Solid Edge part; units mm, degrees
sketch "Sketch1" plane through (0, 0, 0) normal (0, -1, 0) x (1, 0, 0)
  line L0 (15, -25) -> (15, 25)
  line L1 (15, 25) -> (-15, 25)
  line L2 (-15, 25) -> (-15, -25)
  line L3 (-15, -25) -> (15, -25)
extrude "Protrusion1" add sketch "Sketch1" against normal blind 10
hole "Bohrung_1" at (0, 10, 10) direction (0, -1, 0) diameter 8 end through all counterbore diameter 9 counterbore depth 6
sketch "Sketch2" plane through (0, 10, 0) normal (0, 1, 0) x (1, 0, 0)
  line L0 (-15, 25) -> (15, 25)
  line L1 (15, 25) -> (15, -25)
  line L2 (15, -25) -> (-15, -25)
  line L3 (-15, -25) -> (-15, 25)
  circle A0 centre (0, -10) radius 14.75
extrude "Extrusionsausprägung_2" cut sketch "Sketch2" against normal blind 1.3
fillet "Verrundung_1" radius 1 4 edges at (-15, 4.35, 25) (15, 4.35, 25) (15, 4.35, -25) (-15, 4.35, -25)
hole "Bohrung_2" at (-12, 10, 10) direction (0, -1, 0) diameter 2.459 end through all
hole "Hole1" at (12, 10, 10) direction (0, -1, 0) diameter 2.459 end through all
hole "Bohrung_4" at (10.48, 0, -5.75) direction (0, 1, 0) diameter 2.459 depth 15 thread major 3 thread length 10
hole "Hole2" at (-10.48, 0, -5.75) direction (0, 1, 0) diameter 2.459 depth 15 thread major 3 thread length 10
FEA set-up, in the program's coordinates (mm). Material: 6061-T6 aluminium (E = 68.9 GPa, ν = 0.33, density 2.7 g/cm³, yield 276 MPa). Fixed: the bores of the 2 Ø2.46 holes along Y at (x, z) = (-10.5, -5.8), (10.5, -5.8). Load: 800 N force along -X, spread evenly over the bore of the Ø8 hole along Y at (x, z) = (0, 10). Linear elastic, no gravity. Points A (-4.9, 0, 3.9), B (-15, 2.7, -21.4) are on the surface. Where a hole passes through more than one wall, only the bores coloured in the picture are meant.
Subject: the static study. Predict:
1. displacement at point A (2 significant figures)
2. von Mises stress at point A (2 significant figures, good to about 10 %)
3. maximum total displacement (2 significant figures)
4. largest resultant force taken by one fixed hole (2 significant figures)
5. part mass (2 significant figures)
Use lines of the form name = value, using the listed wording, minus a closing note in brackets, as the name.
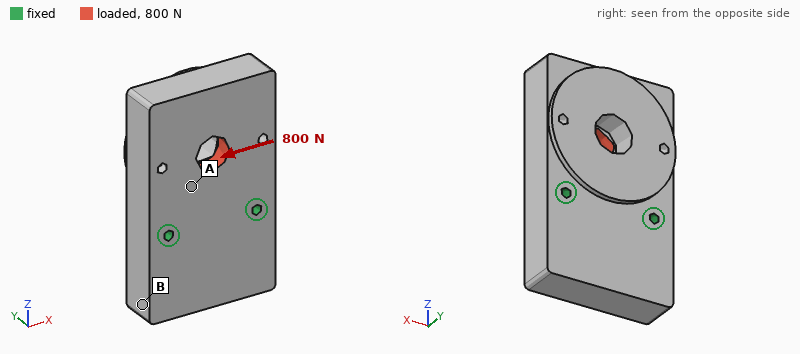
displacement at point A = 2.2 µm
von Mises stress at point A = 9.7 MPa
maximum total displacement = 6.8 µm
largest resultant force taken by one fixed hole = 700 N
part mass = 36 g
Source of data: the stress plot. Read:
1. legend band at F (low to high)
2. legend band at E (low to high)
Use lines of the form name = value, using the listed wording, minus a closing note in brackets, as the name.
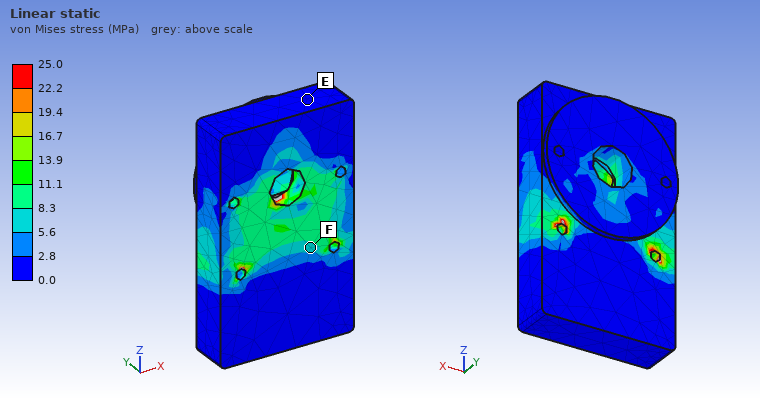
legend band at F = 5.6 to 8.3 MPa
legend band at E = 0.0 to 2.8 MPa
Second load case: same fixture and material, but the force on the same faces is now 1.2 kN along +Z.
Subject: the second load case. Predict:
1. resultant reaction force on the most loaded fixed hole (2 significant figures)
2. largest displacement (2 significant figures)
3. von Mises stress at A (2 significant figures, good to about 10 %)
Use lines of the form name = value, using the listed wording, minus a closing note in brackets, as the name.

resultant reaction force on the most loaded fixed hole = 610 N
largest displacement = 11 µm
von Mises stress at A = 13 MPa
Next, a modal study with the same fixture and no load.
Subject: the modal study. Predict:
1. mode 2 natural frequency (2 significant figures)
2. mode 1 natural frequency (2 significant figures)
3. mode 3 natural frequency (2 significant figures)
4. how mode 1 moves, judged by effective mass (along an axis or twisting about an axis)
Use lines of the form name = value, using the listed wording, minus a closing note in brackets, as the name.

mode 2 natural frequency = 15 kHz
mode 1 natural frequency = 6200 Hz
mode 3 natural frequency = 15 kHz
how mode 1 moves, judged by effective mass = along Y
